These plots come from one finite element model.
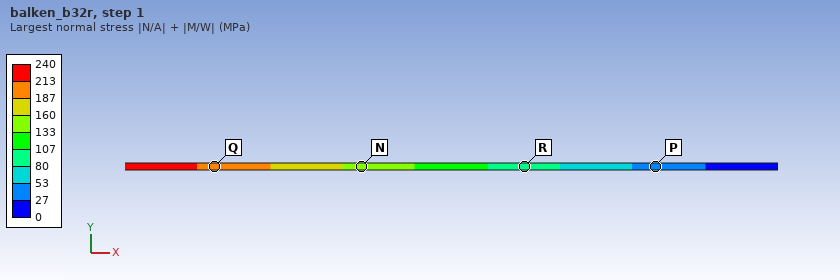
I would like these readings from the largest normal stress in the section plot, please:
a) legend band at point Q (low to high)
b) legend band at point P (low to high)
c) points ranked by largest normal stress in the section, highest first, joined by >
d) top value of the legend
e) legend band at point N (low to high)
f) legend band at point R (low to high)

187 to 213 MPa
27 to 53 MPa
Q > N > R > P
240 MPa
133 to 160 MPa
80 to 107 MPa
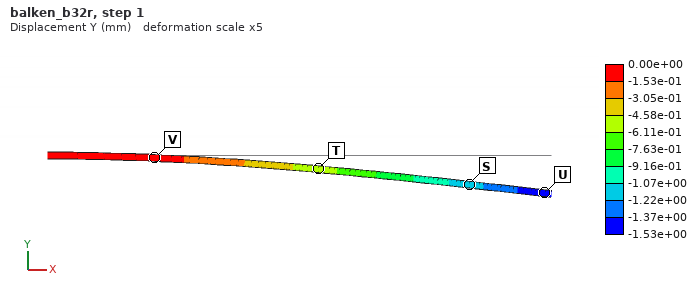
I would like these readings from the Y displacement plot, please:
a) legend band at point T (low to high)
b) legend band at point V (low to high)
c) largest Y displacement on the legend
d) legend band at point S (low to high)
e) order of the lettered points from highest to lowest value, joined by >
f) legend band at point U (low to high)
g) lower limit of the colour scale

-6.11e-01 to -4.58e-01 mm
-1.53e-01 to 0.00e+00 mm
0.00e+00 mm
-1.22e+00 to -1.07e+00 mm
V > T > S > U
-1.53e+00 to -1.37e+00 mm
-1.53e+00 mm
